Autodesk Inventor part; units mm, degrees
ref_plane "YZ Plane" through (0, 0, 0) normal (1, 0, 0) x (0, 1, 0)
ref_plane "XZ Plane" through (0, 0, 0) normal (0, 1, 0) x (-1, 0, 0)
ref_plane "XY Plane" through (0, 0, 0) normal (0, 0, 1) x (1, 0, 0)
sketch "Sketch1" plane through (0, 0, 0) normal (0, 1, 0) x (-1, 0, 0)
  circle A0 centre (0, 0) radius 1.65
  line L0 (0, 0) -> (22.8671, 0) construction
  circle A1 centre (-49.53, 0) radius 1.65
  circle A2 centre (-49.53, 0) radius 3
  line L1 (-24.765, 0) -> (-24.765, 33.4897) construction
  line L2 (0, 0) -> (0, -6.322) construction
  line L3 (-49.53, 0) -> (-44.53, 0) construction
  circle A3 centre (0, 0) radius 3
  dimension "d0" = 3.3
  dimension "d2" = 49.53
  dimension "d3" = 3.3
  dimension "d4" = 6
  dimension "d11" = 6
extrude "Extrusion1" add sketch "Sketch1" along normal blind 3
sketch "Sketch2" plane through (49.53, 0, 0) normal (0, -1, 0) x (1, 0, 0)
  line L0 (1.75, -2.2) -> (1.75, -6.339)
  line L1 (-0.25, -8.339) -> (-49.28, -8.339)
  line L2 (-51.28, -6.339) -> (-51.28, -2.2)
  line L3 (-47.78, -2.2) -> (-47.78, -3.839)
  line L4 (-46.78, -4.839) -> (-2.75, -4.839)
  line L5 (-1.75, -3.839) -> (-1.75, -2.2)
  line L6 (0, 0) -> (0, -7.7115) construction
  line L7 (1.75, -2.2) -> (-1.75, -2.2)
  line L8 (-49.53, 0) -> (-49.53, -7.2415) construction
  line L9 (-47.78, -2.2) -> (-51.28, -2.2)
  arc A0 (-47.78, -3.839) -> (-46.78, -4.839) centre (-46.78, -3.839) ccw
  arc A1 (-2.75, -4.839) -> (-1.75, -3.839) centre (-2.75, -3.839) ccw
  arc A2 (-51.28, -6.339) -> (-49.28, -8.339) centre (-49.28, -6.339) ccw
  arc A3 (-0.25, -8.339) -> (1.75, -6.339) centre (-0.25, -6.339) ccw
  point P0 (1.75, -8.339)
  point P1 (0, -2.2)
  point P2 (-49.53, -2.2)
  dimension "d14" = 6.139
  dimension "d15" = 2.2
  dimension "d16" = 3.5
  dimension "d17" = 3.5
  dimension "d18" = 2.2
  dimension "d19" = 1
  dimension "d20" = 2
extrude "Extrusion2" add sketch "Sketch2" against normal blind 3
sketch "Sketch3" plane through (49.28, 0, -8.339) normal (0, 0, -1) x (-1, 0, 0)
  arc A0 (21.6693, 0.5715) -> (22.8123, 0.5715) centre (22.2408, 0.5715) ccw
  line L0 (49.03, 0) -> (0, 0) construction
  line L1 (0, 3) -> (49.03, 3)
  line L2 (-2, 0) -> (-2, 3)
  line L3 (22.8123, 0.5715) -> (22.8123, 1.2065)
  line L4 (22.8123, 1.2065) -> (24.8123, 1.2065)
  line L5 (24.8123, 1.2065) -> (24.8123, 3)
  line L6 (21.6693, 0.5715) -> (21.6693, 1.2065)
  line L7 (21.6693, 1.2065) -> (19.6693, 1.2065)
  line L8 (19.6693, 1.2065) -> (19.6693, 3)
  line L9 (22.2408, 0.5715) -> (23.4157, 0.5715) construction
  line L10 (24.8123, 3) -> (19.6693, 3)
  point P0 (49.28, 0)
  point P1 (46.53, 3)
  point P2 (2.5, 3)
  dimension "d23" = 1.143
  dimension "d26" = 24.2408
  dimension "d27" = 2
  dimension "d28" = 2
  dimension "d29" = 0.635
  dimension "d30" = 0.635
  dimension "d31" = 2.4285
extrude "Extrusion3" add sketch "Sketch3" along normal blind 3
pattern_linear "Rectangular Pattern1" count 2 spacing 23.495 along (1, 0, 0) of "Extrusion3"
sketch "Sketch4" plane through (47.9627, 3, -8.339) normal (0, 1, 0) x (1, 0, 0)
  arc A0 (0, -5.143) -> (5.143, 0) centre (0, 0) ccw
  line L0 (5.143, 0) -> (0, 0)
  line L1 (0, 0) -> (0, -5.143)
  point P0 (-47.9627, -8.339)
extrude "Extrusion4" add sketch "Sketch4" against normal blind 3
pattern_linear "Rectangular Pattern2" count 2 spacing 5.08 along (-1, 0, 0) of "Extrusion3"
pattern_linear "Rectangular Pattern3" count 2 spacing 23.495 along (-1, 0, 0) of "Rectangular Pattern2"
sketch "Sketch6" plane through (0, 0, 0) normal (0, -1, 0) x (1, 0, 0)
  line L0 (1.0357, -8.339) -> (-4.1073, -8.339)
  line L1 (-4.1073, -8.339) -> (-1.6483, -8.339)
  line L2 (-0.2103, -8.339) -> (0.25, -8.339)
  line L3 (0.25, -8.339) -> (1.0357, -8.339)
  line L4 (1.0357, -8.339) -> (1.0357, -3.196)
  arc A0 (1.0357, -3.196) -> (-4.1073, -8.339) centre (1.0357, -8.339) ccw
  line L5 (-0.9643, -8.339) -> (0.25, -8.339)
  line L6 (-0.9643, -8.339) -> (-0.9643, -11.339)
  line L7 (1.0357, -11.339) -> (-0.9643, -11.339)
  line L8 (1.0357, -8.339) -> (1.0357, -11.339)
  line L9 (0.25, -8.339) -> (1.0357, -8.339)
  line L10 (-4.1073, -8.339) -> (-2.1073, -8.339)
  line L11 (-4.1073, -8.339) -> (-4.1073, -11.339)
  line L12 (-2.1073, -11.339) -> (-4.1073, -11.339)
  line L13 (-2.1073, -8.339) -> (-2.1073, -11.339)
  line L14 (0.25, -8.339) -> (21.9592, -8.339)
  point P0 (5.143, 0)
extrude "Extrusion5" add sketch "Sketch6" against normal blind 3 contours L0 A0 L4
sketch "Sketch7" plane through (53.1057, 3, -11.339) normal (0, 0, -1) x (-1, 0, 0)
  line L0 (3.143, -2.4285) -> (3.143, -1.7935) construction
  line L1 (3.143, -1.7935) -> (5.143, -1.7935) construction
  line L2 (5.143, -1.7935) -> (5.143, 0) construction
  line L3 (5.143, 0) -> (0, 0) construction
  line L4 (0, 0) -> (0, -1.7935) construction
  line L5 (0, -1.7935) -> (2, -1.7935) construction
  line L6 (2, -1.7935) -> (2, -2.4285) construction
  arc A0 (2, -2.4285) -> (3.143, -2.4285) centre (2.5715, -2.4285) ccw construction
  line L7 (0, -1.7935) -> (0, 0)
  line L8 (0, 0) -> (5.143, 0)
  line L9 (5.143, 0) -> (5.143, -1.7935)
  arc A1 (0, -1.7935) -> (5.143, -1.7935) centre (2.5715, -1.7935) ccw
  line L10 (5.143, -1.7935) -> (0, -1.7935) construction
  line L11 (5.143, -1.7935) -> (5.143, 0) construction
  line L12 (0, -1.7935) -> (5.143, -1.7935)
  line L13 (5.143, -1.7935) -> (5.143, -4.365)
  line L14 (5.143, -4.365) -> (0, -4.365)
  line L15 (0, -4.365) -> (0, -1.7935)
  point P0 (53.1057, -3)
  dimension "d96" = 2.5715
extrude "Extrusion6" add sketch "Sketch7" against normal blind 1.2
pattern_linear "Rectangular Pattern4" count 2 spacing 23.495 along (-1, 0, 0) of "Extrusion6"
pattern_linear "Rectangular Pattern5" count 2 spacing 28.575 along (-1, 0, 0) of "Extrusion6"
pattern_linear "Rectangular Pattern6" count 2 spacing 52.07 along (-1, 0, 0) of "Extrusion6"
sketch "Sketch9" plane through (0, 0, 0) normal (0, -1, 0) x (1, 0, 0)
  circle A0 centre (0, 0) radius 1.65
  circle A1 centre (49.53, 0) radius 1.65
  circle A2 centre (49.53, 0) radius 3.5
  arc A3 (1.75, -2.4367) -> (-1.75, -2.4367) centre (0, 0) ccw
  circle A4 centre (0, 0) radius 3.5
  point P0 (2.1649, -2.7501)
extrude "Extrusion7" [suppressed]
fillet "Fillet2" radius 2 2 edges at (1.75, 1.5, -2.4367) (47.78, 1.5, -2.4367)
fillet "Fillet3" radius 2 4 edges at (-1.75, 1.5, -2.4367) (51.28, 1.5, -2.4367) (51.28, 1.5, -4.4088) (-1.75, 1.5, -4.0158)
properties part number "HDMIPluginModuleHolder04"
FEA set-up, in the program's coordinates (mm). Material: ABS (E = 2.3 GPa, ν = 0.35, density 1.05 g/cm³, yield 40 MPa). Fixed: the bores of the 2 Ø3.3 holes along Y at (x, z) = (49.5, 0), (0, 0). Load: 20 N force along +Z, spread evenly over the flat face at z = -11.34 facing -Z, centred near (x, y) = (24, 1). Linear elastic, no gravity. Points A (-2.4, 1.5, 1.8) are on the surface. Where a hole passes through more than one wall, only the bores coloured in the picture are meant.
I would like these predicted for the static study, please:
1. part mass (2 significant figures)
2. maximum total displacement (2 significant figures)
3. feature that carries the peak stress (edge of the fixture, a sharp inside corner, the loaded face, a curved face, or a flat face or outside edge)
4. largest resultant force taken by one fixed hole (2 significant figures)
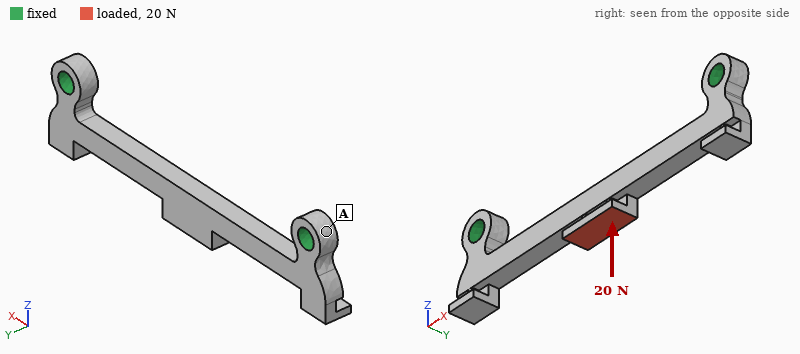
0.99 g
0.46 mm
a curved face
21 N
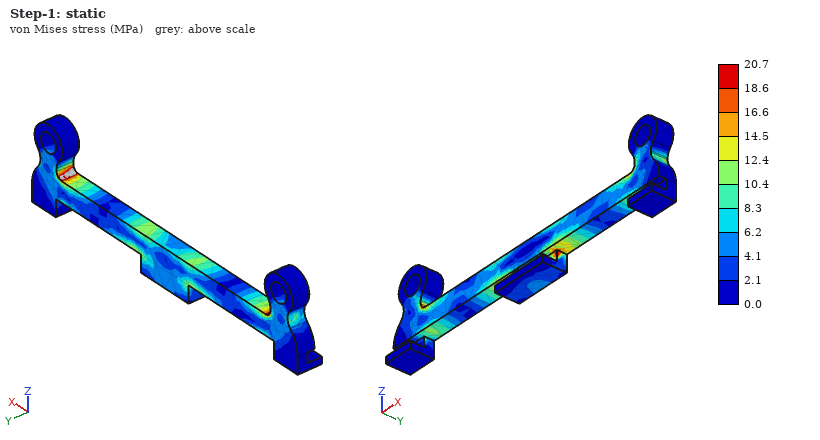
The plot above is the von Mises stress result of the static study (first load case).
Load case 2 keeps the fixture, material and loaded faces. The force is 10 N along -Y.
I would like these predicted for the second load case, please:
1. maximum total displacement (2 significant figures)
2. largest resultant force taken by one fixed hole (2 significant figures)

0.70 mm
5.1 N
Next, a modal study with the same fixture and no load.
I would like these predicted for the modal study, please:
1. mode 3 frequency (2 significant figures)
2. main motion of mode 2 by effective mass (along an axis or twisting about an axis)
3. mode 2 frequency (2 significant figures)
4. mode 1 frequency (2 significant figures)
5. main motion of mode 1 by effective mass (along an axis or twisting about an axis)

3800 Hz
along Z
1900 Hz
1200 Hz
along Y
